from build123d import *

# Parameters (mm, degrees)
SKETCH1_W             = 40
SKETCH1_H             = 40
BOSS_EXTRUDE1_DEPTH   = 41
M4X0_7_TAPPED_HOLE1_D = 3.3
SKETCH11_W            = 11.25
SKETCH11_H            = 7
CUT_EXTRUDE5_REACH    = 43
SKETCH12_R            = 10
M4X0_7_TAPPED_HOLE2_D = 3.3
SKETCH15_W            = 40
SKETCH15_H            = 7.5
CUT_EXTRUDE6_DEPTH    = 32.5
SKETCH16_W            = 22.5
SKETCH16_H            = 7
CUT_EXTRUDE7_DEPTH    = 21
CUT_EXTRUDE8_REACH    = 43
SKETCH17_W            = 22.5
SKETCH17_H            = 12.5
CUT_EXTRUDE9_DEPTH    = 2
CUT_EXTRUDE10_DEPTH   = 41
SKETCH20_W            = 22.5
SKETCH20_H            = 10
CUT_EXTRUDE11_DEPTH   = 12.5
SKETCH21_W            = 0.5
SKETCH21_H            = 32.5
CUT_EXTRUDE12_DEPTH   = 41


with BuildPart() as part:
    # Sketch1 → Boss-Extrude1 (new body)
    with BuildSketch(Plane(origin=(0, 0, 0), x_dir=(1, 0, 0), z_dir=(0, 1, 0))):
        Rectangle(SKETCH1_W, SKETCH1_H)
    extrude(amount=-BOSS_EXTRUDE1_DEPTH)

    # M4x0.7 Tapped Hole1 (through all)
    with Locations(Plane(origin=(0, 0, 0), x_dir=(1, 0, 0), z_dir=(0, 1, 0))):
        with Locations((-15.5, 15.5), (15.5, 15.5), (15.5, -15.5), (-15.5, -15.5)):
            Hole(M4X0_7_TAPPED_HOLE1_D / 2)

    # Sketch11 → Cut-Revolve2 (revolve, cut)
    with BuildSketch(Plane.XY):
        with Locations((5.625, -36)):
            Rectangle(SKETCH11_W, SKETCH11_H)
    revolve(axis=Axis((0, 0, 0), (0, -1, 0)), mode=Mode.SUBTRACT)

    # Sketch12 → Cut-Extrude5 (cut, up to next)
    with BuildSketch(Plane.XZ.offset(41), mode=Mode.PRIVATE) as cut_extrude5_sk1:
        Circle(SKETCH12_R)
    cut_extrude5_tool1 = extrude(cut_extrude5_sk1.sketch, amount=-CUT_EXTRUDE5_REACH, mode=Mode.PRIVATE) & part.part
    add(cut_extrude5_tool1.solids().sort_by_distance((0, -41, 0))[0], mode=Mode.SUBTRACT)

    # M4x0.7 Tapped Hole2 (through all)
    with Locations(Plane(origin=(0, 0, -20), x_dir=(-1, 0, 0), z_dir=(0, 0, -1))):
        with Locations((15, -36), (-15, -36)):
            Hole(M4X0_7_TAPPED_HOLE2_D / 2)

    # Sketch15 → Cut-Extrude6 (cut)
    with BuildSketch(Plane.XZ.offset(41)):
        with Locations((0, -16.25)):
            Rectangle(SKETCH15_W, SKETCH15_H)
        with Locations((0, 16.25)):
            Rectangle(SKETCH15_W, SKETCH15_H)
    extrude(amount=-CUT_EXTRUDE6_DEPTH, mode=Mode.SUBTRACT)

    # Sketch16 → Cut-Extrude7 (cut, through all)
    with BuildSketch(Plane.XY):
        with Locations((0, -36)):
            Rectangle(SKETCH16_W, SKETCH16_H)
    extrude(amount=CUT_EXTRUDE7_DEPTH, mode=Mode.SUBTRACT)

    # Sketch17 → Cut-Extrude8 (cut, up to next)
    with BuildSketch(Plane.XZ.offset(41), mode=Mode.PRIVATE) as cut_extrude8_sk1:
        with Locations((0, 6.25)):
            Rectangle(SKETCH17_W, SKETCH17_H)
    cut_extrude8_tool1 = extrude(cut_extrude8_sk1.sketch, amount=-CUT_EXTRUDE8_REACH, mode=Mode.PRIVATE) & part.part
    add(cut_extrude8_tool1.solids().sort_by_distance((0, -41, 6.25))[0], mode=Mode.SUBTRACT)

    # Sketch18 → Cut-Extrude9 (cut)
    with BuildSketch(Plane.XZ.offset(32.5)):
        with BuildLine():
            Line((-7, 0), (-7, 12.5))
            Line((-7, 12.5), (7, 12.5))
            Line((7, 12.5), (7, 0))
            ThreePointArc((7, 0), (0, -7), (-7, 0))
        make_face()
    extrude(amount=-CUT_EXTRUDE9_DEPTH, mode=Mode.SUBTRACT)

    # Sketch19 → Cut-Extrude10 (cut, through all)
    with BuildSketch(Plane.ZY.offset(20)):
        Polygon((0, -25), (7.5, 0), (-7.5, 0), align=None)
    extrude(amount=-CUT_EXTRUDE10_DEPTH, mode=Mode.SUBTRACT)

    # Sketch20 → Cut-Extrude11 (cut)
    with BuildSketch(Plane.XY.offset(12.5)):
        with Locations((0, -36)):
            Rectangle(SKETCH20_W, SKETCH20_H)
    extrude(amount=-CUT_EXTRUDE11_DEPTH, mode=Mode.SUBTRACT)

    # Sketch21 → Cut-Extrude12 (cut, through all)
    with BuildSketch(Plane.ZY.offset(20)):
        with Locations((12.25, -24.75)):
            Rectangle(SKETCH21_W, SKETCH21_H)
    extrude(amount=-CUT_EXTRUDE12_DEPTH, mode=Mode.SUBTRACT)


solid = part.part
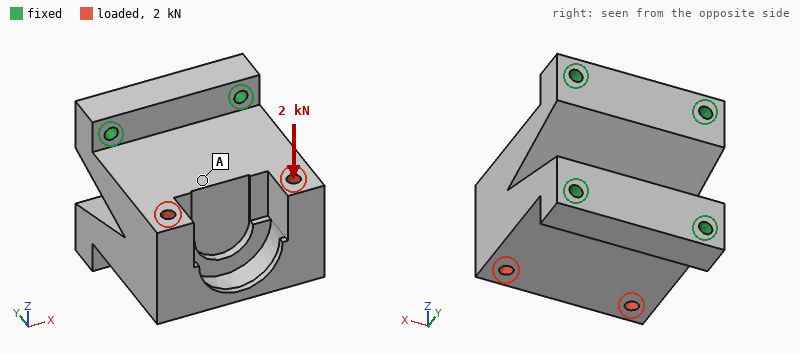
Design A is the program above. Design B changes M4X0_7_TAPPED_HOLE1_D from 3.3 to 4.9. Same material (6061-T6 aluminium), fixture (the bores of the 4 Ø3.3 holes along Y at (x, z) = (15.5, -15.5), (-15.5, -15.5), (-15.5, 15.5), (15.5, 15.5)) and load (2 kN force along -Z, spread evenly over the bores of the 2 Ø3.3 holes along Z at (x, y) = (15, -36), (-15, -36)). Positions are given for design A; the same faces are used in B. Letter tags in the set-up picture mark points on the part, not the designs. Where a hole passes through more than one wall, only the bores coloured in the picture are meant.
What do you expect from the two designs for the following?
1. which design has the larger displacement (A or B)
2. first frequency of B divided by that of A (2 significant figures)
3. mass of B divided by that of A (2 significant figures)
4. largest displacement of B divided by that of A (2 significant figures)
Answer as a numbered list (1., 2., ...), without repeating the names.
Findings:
1. A
2. 1.1
3. 0.99
4. 0.89
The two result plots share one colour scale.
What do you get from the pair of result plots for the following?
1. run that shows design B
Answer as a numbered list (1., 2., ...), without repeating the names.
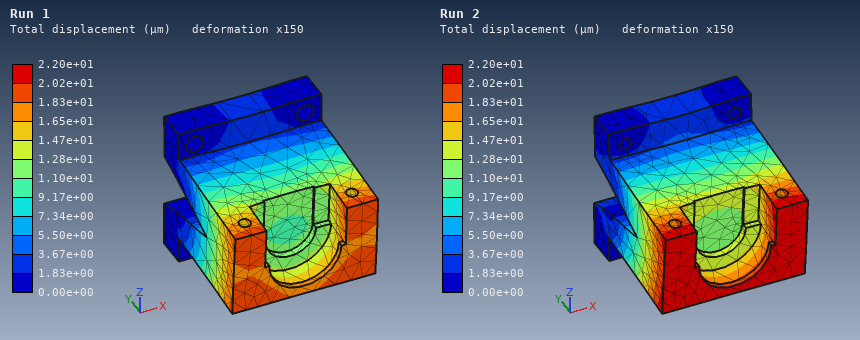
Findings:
1. Run 1
